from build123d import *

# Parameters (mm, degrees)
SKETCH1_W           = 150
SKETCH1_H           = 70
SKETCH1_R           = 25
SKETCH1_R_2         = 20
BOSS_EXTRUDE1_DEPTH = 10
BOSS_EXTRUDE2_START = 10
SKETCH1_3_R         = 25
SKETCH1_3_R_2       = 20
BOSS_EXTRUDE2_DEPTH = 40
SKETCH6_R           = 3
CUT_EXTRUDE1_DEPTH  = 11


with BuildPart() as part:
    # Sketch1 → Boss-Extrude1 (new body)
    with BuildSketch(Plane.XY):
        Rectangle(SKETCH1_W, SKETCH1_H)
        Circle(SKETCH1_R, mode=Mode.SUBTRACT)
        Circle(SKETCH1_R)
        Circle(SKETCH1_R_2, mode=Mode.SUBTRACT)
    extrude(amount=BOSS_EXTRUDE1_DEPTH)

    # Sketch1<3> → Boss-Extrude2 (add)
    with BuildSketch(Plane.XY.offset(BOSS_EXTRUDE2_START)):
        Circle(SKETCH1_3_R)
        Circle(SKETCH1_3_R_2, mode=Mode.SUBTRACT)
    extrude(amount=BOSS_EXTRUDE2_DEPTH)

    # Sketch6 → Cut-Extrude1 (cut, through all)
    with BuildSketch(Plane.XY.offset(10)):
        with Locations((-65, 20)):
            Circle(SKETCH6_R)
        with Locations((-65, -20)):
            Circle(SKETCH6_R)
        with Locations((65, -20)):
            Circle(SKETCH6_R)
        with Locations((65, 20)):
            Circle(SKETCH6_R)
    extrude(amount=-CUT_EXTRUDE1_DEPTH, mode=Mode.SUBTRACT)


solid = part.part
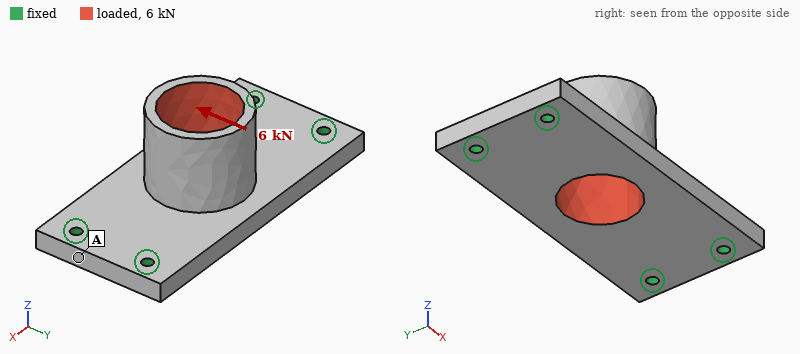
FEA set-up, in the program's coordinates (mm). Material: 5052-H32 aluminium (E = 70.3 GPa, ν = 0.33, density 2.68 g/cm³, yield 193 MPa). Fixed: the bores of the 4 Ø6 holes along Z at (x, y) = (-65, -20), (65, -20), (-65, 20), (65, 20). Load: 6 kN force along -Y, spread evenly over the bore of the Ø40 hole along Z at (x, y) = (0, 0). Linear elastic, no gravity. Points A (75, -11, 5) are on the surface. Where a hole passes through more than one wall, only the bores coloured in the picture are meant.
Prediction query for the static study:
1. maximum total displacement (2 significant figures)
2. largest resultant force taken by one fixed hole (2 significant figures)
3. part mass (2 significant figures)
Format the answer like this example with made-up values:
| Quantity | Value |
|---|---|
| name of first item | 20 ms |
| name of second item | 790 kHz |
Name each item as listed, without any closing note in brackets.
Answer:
| Quantity | Value |
|---|---|
| maximum total displacement | 0.20 mm |
| largest resultant force taken by one fixed hole | 2.7 kN |
| part mass | 320 g |
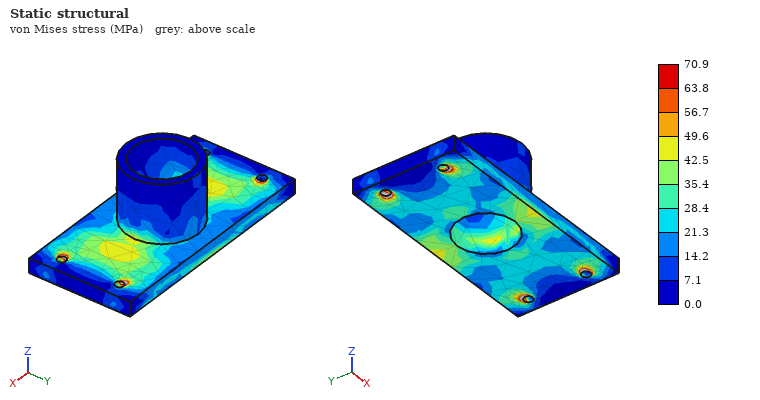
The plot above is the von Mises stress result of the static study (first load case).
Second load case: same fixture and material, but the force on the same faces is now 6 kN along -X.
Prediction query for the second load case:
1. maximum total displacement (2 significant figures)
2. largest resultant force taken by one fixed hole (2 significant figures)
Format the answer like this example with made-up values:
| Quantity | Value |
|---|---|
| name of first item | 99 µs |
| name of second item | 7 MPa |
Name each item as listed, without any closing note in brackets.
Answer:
| Quantity | Value |
|---|---|
| maximum total displacement | 72 µm |
| largest resultant force taken by one fixed hole | 1.6 kN |
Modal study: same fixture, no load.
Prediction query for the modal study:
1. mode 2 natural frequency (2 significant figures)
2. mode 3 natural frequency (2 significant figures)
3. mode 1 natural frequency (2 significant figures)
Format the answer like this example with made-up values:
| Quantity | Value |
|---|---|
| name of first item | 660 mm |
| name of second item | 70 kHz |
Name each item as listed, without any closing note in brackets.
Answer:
| Quantity | Value |
|---|---|
| mode 2 natural frequency | 2700 Hz |
| mode 3 natural frequency | 4600 Hz |
| mode 1 natural frequency | 2700 Hz |
